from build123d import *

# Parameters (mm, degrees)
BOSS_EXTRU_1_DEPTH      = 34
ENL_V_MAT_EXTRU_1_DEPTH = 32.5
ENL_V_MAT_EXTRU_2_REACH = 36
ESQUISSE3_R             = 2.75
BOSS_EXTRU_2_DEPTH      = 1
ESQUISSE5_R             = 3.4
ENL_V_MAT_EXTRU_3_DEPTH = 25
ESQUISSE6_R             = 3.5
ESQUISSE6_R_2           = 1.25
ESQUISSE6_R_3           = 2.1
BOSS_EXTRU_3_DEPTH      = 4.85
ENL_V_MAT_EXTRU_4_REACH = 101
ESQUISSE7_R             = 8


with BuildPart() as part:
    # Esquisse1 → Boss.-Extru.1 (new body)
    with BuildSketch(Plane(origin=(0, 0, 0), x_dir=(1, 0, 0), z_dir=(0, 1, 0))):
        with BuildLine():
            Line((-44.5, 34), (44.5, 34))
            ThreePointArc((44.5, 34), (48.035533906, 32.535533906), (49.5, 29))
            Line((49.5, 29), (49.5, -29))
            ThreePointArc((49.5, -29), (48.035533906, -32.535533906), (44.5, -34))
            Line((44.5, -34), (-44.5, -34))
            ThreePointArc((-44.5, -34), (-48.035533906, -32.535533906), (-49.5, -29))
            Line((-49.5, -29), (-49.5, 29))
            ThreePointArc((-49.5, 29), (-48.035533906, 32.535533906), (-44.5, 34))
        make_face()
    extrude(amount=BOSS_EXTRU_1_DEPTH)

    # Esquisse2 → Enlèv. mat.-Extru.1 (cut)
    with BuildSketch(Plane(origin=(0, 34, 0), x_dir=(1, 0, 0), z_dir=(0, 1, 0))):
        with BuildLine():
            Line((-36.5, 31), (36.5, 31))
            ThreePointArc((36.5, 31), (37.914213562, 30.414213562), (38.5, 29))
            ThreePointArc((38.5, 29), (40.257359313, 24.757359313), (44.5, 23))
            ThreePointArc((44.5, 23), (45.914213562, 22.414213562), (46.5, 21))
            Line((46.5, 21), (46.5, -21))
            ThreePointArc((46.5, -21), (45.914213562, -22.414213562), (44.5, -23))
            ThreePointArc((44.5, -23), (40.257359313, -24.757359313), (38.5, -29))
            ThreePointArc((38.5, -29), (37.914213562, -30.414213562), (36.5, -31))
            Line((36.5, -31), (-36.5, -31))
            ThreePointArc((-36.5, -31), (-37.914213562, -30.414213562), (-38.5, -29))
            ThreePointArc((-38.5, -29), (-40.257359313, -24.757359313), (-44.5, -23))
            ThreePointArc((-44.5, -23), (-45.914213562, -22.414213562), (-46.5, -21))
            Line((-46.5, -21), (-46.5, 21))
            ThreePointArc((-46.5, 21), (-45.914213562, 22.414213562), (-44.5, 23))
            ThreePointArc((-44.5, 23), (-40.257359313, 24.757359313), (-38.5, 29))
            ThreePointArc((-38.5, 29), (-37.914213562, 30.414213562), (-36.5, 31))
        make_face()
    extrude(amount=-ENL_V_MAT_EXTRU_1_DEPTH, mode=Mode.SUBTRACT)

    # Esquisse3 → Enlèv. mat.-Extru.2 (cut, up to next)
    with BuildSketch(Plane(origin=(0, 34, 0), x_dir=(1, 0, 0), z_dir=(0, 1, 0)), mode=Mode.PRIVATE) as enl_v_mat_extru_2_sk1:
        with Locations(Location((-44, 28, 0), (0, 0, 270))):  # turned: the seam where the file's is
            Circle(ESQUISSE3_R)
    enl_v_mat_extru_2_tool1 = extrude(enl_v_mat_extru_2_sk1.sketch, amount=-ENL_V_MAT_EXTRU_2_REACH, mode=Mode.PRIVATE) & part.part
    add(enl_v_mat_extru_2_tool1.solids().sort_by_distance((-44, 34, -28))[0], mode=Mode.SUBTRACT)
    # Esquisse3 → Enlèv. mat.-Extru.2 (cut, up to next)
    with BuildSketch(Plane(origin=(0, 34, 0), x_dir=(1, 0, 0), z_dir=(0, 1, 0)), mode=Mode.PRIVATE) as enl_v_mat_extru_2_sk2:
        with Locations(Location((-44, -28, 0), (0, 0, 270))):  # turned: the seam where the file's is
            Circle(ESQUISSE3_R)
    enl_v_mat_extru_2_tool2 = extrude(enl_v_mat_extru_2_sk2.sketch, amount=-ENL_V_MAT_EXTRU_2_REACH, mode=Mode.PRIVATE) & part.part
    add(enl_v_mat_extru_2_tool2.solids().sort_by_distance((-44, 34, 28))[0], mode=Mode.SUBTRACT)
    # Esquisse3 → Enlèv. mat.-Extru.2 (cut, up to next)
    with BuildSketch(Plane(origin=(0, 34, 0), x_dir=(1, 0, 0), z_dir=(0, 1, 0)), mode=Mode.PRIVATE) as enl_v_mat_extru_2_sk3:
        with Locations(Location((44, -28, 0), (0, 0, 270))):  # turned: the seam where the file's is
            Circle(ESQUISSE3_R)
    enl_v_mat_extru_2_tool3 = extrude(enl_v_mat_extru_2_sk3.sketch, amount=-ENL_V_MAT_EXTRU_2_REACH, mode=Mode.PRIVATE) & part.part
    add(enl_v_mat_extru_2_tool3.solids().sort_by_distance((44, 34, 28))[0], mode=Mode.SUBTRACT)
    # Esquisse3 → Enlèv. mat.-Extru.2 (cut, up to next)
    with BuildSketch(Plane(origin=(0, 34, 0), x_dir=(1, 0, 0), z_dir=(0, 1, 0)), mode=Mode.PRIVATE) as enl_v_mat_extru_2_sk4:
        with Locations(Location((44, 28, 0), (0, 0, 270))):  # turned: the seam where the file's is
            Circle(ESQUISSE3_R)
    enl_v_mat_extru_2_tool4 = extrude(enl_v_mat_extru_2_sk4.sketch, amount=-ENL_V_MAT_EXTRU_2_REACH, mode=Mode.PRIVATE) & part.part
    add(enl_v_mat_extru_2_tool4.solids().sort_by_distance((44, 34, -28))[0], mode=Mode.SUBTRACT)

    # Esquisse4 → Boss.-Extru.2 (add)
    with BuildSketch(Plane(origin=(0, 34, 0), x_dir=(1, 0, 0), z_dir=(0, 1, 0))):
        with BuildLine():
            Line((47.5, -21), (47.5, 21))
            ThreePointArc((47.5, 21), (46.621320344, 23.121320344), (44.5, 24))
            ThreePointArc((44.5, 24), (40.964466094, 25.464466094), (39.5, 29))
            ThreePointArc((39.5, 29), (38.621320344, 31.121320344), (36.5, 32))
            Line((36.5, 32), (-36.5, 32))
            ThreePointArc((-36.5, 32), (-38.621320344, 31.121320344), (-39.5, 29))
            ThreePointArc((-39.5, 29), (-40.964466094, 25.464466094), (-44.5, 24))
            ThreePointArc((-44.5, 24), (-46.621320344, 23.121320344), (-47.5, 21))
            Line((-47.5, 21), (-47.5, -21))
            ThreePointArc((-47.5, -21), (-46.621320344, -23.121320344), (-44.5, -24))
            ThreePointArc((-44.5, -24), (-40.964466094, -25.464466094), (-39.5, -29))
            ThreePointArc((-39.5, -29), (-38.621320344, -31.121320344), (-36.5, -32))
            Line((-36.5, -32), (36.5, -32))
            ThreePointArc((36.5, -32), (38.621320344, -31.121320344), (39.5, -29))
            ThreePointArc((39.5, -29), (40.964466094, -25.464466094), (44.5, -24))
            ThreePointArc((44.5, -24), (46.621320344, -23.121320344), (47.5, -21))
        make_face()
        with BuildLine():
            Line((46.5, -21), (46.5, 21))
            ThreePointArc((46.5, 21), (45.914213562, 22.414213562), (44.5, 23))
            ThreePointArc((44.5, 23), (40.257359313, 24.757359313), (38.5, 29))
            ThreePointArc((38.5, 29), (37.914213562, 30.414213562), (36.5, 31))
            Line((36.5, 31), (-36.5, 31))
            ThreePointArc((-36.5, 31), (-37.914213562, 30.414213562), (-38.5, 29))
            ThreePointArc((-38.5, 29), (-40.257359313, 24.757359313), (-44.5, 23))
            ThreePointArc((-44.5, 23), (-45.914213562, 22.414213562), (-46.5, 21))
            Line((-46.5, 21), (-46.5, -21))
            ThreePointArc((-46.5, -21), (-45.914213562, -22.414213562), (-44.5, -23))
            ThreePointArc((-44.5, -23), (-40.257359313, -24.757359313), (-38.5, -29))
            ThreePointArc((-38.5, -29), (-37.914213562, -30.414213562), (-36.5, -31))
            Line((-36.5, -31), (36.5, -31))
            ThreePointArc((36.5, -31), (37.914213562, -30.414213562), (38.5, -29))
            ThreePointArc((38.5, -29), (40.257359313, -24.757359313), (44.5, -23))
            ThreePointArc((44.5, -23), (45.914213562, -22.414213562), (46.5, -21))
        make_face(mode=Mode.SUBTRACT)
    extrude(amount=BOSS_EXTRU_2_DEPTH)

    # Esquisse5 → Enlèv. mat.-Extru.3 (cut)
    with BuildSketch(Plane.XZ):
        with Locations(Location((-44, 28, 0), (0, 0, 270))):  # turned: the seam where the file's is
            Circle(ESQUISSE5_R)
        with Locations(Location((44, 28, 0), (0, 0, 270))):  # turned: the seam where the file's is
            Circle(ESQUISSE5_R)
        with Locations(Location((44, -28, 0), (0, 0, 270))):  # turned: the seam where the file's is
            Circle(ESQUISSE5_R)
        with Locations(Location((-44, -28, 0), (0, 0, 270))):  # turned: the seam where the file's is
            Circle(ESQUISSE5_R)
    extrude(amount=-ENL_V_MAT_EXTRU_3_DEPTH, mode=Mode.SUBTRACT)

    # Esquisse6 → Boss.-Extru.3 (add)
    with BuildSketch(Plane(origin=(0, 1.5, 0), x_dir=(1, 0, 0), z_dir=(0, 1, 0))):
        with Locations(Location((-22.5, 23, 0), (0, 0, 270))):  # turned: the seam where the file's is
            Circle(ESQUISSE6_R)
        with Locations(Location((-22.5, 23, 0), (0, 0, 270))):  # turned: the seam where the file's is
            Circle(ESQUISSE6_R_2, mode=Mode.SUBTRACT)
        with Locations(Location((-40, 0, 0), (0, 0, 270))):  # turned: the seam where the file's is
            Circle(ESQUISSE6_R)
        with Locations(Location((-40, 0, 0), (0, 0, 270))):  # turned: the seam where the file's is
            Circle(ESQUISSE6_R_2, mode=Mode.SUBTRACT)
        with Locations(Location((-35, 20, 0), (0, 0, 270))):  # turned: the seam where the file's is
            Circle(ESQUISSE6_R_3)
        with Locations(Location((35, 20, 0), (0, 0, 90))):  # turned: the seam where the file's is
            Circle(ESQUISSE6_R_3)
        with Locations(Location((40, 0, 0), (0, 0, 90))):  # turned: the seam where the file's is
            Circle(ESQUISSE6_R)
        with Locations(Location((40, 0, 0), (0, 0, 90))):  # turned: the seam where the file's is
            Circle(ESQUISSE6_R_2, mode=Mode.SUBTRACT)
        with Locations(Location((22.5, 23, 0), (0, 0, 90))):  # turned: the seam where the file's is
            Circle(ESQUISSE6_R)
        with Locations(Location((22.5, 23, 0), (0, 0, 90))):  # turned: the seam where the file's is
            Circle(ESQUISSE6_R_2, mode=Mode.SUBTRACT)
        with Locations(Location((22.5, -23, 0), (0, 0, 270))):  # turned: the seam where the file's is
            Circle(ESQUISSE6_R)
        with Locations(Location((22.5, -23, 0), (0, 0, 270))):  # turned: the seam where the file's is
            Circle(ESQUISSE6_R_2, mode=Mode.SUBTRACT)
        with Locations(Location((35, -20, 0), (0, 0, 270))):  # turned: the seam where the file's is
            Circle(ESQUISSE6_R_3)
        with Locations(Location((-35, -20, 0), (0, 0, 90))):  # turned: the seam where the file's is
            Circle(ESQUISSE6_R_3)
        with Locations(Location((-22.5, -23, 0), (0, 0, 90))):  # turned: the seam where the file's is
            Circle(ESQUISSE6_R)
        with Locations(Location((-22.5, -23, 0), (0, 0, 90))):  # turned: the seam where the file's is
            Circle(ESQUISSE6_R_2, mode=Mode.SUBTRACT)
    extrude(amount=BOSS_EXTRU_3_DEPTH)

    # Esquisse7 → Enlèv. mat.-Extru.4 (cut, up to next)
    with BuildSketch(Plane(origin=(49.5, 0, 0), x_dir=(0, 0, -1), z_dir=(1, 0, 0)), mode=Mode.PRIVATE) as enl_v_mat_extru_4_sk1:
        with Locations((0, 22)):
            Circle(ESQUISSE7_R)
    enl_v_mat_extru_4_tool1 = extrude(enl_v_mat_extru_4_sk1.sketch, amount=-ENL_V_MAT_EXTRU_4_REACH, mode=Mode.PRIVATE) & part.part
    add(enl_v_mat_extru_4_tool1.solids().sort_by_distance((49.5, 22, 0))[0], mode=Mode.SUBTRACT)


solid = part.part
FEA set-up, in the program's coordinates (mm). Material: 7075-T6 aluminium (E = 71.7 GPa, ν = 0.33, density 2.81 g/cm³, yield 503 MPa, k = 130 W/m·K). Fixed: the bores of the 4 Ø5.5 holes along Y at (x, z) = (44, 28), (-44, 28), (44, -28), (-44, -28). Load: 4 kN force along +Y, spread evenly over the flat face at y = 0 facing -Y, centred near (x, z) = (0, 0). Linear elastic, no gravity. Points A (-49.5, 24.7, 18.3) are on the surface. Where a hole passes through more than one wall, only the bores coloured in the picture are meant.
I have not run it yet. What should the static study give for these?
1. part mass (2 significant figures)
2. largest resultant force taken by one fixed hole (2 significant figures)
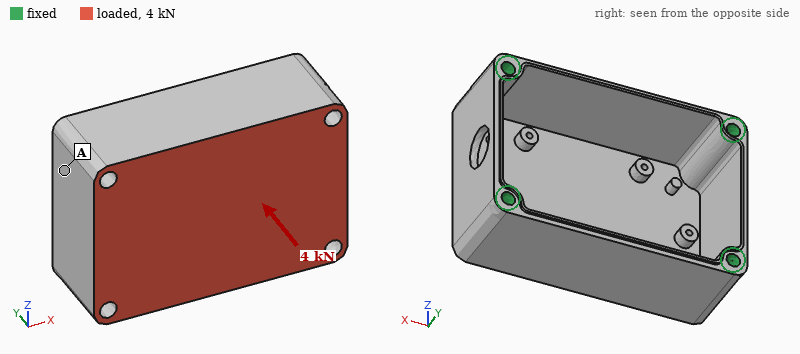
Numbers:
130 g
1.1 kN
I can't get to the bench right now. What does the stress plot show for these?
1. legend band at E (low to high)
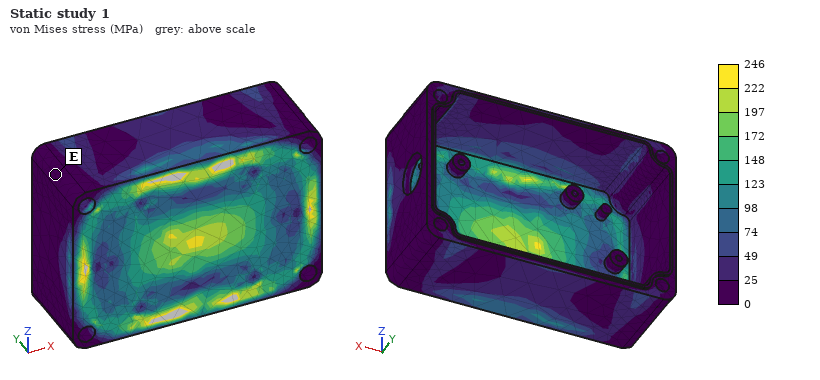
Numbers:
0 to 25 MPa
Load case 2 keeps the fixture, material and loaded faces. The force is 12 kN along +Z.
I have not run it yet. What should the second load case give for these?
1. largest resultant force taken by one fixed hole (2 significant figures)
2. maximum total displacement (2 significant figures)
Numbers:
4.2 kN
0.12 mm
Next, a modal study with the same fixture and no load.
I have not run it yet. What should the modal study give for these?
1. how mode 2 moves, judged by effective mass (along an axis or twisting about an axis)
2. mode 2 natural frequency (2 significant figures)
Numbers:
along Z
3200 Hz
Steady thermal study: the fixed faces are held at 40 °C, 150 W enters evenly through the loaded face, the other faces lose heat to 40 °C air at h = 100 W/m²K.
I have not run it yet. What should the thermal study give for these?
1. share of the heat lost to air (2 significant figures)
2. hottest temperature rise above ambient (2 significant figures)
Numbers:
48 %
67 K
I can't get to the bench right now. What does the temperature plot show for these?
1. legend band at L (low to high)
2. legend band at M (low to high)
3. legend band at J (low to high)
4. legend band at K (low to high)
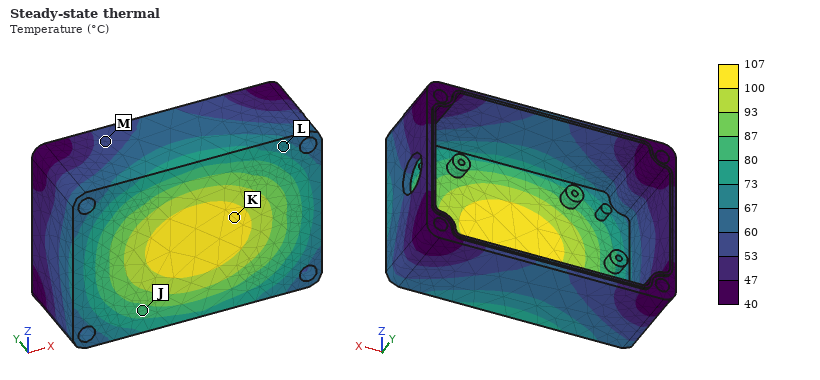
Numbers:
67 to 73 °C
53 to 60 °C
80 to 87 °C
100 to 107 °C
